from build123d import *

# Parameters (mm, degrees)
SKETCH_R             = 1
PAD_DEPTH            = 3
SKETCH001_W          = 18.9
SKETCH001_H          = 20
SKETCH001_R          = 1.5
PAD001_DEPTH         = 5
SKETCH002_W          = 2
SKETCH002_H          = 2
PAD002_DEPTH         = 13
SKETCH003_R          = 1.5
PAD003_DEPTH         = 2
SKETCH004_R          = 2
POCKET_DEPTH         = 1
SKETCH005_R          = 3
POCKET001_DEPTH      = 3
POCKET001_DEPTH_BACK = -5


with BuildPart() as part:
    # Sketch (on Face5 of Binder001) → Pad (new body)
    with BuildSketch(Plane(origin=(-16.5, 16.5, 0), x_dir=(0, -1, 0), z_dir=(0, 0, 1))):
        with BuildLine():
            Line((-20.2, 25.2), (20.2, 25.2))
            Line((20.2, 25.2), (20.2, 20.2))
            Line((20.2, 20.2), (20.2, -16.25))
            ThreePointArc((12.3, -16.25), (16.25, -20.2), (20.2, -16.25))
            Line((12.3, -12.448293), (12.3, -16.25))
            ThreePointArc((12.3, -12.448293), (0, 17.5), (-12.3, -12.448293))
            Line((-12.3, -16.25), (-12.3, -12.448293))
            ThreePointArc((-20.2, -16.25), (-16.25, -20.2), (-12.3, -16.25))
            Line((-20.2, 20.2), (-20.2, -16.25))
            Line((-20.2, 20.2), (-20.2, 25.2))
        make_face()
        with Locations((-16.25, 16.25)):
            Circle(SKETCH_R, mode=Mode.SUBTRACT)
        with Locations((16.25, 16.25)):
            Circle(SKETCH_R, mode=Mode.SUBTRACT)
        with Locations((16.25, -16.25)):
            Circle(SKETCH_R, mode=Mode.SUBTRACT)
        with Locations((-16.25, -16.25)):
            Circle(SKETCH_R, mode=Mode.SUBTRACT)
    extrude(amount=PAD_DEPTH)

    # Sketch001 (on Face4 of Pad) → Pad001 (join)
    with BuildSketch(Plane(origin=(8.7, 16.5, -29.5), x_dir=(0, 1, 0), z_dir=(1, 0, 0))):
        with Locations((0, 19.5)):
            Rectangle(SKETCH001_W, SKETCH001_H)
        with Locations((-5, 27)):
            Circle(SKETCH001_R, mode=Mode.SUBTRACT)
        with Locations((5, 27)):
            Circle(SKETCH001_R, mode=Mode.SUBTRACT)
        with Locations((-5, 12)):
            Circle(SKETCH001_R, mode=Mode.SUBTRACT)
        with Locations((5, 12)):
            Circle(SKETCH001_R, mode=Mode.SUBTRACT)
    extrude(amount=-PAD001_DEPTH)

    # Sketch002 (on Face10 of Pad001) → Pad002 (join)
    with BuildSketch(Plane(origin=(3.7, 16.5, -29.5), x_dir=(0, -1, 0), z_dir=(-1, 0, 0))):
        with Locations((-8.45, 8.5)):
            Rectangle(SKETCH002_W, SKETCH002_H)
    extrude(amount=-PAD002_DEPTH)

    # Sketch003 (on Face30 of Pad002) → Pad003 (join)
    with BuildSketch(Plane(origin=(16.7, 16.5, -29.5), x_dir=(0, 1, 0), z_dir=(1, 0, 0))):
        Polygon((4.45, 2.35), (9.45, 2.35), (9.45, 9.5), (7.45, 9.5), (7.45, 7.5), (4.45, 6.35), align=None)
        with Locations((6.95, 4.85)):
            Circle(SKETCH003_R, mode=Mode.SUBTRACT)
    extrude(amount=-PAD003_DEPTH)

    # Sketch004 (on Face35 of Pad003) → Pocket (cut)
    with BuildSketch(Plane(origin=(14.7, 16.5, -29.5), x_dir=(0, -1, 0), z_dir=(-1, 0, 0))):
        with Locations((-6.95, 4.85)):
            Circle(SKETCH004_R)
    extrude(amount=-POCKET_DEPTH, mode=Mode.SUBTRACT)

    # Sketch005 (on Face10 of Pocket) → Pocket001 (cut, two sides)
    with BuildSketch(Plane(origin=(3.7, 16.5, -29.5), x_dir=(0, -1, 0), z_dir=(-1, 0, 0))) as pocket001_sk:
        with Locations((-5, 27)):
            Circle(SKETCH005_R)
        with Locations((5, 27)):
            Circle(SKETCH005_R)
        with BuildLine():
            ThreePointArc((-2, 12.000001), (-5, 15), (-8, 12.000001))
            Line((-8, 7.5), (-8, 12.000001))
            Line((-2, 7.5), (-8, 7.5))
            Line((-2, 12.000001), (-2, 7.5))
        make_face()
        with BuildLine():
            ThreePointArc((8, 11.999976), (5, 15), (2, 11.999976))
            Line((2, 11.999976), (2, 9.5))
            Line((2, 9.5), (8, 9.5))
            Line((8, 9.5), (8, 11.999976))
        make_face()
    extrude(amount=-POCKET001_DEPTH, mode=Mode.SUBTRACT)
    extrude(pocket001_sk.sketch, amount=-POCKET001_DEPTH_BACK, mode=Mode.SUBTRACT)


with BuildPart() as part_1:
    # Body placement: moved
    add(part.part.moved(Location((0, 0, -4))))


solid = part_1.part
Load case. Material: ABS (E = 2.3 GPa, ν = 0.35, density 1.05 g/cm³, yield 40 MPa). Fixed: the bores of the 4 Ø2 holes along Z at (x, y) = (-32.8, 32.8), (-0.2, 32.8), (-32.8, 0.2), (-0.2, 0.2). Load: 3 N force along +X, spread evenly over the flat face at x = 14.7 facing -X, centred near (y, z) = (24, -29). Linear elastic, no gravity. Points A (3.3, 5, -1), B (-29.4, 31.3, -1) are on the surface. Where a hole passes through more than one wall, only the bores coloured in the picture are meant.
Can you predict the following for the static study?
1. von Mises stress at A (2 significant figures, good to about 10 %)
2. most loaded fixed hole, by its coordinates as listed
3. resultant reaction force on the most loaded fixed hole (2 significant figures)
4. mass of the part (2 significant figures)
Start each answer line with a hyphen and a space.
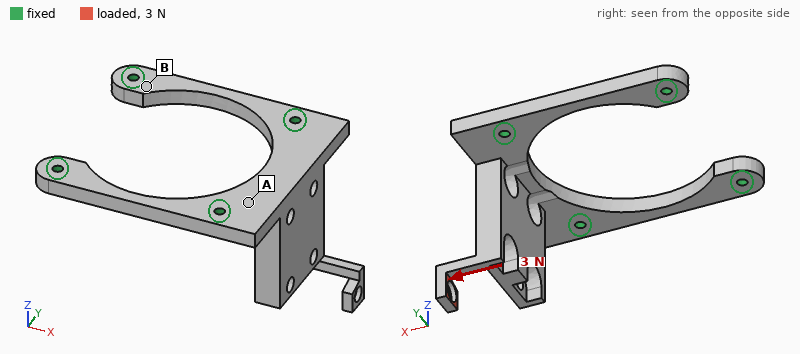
- 2.0 MPa
- (-0.2, 32.8)
- 2.8 N
- 4.0 g
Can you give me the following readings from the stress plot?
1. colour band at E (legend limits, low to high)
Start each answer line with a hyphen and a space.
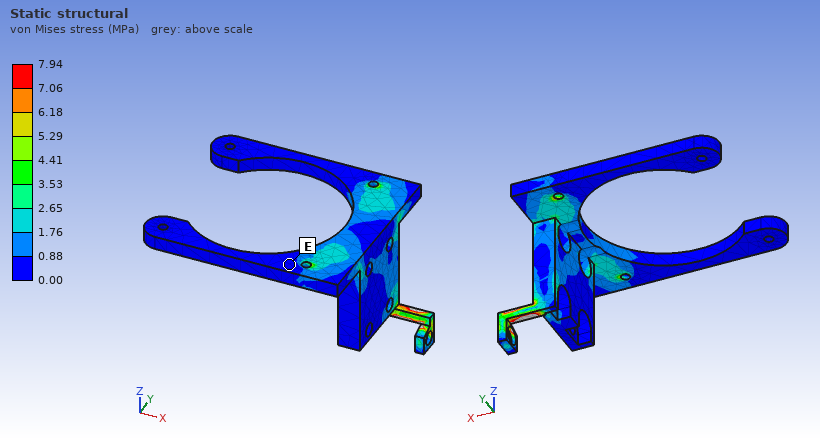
- 0.00 to 0.88 MPa
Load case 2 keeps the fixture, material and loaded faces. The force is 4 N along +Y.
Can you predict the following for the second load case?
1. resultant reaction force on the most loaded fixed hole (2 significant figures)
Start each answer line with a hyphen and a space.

- 4.9 N
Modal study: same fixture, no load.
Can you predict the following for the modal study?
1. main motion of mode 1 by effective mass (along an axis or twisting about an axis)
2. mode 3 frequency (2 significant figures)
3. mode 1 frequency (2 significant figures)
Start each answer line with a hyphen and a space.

- along X
- 2300 Hz
- 860 Hz
